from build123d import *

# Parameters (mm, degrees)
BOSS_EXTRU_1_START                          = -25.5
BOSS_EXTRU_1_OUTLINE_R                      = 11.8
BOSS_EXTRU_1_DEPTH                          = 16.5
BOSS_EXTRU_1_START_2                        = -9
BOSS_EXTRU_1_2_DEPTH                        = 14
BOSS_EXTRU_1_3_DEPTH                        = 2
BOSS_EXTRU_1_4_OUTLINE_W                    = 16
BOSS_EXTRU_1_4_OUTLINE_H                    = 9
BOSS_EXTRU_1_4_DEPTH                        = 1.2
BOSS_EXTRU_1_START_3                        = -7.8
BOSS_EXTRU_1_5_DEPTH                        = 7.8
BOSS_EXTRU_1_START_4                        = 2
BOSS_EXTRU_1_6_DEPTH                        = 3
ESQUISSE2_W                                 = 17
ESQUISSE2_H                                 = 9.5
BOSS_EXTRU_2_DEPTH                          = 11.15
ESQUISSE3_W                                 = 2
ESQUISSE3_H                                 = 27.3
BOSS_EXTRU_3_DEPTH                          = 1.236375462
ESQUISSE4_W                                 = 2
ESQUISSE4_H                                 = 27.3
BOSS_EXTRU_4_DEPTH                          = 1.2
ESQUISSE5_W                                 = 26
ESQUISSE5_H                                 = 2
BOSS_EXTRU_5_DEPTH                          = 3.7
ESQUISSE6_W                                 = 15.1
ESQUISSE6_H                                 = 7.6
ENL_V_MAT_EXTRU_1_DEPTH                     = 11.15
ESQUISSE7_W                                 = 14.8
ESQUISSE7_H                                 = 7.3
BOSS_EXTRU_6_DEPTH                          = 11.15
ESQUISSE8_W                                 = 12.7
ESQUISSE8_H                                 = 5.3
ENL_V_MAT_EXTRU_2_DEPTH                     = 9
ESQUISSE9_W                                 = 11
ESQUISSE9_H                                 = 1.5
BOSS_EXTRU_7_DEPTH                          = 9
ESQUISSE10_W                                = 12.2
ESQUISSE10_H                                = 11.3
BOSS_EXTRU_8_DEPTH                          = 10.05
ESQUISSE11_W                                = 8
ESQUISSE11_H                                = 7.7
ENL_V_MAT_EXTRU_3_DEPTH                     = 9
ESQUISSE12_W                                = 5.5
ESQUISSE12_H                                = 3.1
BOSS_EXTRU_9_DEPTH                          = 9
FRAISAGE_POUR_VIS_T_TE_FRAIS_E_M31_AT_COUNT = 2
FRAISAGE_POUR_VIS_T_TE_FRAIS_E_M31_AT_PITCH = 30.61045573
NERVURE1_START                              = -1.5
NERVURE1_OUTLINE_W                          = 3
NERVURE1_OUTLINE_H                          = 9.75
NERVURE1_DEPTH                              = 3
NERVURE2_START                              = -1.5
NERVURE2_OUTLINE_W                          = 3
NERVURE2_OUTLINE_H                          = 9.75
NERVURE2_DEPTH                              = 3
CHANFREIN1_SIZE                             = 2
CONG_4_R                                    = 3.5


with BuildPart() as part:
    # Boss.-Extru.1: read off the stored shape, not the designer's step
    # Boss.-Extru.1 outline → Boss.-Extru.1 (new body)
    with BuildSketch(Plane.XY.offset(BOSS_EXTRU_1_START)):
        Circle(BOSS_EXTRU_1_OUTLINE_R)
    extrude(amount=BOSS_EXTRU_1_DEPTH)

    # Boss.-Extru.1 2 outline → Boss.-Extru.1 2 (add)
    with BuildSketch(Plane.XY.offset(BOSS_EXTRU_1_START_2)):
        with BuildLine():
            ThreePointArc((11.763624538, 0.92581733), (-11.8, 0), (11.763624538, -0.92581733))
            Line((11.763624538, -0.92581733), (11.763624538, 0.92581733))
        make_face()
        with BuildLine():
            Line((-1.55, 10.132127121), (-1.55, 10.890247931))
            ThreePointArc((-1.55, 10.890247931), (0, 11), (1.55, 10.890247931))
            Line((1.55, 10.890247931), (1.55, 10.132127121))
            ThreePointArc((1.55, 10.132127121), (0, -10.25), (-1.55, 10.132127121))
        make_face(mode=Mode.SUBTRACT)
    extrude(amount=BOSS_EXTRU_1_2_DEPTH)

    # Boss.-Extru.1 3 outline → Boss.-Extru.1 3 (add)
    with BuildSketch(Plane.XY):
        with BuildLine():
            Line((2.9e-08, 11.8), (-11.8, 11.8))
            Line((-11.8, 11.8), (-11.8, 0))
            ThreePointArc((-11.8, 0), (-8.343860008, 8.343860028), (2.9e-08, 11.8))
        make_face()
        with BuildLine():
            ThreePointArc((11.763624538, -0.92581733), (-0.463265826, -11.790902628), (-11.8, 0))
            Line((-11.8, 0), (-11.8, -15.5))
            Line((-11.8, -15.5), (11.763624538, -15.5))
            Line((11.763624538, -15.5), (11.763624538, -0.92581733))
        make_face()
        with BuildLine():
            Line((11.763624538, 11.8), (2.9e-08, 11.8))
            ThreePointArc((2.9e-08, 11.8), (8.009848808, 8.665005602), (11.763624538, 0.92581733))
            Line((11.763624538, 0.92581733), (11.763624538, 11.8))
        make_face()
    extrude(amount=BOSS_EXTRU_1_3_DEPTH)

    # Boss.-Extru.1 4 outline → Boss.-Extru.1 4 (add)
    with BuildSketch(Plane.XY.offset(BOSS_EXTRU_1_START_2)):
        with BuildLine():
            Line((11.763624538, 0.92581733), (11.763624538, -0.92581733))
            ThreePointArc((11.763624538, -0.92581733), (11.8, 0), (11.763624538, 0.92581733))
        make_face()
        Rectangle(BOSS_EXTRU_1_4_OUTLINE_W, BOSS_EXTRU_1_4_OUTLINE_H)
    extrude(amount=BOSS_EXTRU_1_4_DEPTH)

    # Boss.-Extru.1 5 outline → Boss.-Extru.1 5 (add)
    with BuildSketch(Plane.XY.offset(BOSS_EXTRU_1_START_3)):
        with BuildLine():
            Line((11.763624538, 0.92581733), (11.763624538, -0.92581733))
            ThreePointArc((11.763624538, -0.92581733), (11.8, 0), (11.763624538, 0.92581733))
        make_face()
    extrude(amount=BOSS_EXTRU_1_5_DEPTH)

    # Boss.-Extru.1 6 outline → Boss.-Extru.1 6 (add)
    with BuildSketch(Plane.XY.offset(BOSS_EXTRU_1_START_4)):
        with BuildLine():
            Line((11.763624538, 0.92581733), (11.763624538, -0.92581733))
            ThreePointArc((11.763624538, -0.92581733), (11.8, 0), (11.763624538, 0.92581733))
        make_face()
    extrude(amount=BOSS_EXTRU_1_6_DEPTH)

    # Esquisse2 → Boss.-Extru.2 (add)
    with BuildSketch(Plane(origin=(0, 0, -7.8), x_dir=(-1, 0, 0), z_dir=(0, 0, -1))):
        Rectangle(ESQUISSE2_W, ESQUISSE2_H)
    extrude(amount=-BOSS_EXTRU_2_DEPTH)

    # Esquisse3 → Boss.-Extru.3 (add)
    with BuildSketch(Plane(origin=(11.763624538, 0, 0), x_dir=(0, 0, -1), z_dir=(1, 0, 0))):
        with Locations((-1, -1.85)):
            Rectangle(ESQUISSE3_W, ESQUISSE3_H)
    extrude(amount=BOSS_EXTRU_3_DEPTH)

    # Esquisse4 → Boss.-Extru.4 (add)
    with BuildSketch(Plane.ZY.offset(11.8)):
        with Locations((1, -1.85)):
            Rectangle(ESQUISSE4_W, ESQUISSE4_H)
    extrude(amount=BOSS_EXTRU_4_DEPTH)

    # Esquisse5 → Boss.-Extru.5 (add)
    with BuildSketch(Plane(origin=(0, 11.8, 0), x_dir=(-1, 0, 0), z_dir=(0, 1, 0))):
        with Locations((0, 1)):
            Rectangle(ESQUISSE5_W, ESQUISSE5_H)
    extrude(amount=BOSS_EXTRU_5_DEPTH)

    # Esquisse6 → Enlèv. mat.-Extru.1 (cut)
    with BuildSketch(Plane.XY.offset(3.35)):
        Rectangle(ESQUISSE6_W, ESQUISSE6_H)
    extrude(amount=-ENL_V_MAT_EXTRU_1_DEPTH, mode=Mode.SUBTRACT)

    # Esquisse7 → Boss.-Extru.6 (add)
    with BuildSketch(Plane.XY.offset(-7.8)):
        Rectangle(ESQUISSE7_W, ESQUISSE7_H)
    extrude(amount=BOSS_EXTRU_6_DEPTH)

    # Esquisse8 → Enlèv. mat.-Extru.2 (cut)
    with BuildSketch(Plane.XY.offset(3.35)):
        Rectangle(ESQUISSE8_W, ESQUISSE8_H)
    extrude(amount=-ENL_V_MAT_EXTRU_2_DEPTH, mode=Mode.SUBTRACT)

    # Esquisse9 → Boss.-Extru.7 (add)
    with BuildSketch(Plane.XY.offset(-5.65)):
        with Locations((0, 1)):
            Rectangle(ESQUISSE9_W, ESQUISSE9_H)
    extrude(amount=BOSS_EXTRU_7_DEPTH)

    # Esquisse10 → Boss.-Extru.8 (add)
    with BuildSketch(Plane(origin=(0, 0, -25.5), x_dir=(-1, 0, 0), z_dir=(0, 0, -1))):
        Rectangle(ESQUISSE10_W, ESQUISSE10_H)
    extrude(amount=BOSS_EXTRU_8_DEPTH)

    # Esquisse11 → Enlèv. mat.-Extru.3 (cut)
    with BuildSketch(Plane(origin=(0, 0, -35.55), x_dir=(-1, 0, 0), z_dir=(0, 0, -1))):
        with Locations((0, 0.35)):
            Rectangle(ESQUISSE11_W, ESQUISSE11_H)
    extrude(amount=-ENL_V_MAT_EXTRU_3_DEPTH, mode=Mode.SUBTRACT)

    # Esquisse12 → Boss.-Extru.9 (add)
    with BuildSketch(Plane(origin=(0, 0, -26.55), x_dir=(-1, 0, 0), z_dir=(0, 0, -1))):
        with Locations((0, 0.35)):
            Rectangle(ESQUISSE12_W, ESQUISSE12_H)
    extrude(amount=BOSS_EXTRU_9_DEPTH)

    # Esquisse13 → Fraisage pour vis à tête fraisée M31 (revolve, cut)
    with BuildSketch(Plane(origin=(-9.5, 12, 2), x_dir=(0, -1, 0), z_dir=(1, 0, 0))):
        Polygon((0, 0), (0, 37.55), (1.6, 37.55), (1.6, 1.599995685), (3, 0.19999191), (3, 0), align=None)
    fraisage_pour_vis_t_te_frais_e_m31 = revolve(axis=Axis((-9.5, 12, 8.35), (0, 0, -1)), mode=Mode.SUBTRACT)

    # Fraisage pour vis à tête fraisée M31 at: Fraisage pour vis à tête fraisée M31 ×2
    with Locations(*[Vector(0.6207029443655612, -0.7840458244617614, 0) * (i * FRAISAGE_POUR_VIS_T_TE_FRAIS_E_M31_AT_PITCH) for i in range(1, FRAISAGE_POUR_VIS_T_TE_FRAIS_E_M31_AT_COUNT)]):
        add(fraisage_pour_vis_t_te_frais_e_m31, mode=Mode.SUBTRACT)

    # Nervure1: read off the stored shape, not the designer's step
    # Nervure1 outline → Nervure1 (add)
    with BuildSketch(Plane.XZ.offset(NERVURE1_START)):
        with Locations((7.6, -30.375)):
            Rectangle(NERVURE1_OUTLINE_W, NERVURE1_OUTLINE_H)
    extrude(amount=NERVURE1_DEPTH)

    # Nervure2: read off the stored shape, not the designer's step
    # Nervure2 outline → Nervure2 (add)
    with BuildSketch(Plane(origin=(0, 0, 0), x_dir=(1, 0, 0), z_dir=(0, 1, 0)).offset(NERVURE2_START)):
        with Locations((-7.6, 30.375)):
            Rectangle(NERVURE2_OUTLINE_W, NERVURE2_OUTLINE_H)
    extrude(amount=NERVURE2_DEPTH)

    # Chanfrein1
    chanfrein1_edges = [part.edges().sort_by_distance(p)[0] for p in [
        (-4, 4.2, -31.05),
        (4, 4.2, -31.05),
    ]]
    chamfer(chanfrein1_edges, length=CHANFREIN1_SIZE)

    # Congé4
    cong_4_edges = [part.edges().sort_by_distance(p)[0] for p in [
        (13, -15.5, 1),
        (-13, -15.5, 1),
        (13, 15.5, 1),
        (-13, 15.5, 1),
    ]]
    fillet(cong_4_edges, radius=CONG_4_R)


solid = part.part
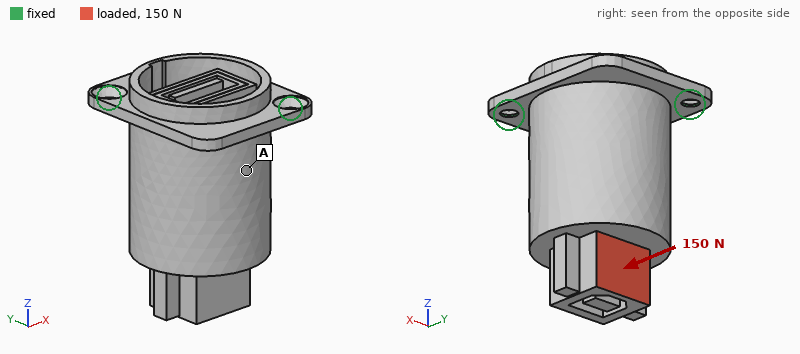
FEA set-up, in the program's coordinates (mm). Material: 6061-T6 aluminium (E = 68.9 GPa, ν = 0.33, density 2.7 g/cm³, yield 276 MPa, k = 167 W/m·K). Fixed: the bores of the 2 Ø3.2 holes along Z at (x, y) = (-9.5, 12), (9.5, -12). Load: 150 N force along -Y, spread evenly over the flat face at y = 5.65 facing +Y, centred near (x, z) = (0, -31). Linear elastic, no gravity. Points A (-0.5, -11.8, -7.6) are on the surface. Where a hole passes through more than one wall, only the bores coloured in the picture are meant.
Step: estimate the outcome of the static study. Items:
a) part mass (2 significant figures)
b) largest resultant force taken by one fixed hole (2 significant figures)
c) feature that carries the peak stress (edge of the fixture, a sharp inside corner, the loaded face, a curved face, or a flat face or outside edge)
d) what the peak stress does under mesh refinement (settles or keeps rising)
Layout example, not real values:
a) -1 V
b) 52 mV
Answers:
a) 32 g
b) 150 N
c) edge of the fixture
d) keeps rising
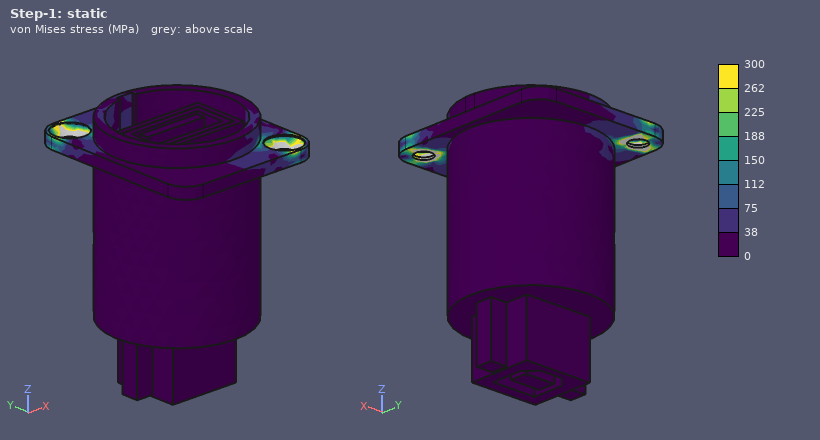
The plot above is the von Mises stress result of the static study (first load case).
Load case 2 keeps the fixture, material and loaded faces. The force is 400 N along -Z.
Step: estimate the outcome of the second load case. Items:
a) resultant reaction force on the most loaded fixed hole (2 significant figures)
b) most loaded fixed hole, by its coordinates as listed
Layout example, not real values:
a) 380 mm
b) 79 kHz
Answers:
a) 260 N
b) (-9.5, 12)
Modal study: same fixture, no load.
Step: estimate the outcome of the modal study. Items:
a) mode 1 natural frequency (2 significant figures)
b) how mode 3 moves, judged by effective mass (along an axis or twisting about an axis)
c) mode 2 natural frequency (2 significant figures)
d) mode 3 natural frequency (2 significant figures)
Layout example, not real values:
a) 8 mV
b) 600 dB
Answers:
a) 620 Hz
b) along Z
c) 3200 Hz
d) 4900 Hz
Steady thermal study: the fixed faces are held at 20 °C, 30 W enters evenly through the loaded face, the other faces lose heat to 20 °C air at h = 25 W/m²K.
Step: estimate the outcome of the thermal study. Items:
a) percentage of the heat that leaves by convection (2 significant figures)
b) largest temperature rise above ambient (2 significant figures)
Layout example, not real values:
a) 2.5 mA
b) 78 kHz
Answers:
a) 24 %
b) 68 K
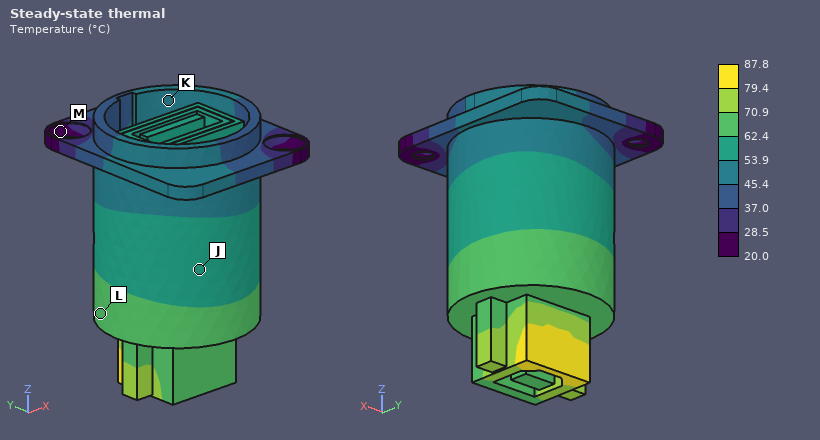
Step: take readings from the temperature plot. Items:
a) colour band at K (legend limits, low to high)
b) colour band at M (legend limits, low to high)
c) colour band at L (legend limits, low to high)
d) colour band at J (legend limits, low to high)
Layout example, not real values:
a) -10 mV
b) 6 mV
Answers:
a) 45.4 to 53.9 °C
b) 20.0 to 28.5 °C
c) 62.4 to 70.9 °C
d) 53.9 to 62.4 °C
